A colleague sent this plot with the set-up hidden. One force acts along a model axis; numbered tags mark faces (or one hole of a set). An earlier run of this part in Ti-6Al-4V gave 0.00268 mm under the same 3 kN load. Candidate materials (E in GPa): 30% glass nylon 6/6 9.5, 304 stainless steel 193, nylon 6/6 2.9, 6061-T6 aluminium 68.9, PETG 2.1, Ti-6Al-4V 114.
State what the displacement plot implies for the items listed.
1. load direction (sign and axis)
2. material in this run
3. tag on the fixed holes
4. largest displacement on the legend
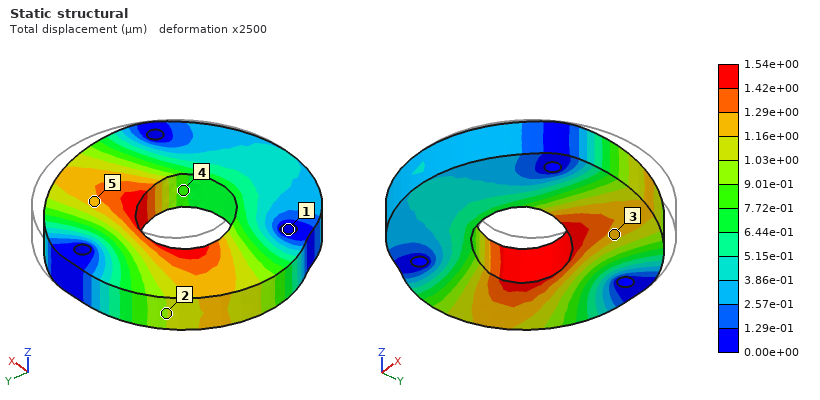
-X
304 stainless steel
1
1.54e+00 µm
